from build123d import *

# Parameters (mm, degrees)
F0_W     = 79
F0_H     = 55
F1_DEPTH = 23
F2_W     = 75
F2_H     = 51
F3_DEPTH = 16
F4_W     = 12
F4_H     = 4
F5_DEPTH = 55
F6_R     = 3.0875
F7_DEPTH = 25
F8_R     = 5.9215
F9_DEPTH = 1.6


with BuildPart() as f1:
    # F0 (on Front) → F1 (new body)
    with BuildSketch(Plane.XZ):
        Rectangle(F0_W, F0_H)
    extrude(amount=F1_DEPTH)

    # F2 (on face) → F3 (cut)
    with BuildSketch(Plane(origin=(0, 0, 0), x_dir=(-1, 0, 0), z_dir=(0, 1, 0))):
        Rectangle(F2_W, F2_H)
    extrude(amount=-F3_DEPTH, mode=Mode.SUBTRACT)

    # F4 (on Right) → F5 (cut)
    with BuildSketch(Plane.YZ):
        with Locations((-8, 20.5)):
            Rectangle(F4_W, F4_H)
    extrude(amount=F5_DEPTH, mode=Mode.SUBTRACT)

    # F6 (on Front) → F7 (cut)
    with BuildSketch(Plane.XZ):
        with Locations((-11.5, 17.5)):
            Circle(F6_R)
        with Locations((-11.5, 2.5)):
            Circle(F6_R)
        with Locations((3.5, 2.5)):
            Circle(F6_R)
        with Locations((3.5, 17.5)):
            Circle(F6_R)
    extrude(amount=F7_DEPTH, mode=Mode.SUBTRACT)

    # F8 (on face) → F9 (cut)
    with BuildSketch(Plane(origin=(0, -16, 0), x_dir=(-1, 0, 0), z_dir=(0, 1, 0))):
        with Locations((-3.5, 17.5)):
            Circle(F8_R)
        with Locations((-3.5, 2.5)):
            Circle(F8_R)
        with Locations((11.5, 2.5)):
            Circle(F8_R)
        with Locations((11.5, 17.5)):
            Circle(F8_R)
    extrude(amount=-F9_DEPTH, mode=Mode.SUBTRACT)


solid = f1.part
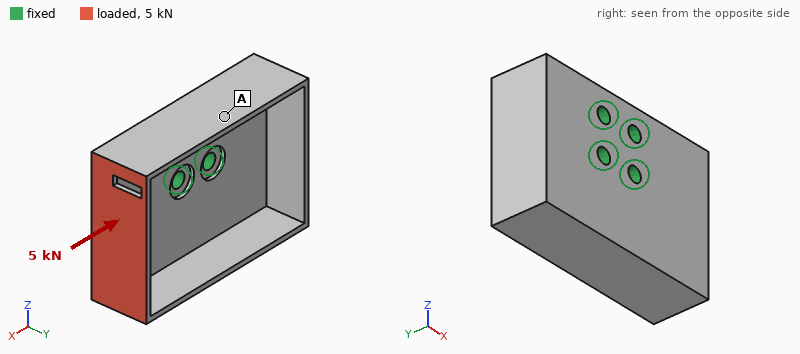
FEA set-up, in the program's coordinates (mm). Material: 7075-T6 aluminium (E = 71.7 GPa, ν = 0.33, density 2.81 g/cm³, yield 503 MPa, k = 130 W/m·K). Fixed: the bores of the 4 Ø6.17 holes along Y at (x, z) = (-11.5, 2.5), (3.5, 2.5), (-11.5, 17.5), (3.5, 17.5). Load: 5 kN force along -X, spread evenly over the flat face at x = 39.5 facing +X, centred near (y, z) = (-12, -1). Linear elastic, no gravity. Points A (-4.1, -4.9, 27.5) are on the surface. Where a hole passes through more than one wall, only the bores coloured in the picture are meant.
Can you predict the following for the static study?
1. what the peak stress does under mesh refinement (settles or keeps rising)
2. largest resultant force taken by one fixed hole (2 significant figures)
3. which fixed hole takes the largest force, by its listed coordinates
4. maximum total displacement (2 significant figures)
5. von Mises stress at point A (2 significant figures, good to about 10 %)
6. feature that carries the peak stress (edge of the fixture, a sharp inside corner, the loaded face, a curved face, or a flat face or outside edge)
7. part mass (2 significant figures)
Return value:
keeps rising
3.1 kN
(3.5, 2.5)
0.67 mm
34 MPa
a sharp inside corner
100 g
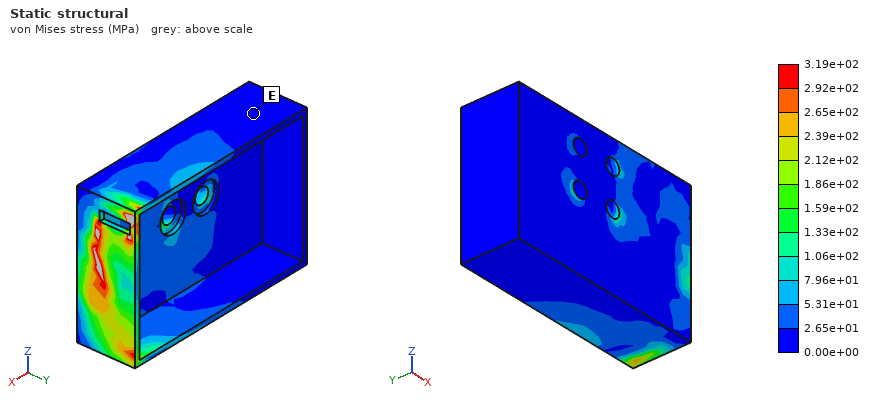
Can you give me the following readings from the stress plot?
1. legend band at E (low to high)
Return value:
0.00e+00 to 2.65e+01 MPa
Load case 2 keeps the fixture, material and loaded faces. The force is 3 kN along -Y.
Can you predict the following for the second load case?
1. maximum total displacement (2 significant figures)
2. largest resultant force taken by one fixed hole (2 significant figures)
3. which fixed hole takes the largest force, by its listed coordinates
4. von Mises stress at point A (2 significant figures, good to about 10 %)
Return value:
0.47 mm
4.5 kN
(3.5, 2.5)
61 MPa
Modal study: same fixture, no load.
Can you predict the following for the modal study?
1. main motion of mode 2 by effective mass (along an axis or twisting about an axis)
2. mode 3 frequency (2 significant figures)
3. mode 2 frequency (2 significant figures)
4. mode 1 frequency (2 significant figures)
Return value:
along Y
5300 Hz
3800 Hz
2900 Hz
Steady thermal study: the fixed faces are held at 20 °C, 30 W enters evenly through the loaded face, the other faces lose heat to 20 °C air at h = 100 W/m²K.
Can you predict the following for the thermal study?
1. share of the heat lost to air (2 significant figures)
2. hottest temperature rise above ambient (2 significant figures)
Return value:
32 %
28 K
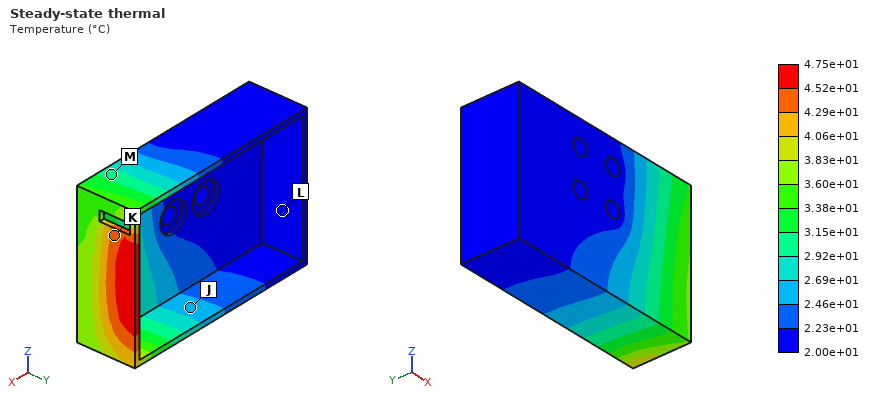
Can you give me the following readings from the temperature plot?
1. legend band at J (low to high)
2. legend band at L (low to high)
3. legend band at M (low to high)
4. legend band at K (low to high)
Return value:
2.46e+01 to 2.69e+01 °C
2.00e+01 to 2.23e+01 °C
2.92e+01 to 3.15e+01 °C
4.29e+01 to 4.52e+01 °C
